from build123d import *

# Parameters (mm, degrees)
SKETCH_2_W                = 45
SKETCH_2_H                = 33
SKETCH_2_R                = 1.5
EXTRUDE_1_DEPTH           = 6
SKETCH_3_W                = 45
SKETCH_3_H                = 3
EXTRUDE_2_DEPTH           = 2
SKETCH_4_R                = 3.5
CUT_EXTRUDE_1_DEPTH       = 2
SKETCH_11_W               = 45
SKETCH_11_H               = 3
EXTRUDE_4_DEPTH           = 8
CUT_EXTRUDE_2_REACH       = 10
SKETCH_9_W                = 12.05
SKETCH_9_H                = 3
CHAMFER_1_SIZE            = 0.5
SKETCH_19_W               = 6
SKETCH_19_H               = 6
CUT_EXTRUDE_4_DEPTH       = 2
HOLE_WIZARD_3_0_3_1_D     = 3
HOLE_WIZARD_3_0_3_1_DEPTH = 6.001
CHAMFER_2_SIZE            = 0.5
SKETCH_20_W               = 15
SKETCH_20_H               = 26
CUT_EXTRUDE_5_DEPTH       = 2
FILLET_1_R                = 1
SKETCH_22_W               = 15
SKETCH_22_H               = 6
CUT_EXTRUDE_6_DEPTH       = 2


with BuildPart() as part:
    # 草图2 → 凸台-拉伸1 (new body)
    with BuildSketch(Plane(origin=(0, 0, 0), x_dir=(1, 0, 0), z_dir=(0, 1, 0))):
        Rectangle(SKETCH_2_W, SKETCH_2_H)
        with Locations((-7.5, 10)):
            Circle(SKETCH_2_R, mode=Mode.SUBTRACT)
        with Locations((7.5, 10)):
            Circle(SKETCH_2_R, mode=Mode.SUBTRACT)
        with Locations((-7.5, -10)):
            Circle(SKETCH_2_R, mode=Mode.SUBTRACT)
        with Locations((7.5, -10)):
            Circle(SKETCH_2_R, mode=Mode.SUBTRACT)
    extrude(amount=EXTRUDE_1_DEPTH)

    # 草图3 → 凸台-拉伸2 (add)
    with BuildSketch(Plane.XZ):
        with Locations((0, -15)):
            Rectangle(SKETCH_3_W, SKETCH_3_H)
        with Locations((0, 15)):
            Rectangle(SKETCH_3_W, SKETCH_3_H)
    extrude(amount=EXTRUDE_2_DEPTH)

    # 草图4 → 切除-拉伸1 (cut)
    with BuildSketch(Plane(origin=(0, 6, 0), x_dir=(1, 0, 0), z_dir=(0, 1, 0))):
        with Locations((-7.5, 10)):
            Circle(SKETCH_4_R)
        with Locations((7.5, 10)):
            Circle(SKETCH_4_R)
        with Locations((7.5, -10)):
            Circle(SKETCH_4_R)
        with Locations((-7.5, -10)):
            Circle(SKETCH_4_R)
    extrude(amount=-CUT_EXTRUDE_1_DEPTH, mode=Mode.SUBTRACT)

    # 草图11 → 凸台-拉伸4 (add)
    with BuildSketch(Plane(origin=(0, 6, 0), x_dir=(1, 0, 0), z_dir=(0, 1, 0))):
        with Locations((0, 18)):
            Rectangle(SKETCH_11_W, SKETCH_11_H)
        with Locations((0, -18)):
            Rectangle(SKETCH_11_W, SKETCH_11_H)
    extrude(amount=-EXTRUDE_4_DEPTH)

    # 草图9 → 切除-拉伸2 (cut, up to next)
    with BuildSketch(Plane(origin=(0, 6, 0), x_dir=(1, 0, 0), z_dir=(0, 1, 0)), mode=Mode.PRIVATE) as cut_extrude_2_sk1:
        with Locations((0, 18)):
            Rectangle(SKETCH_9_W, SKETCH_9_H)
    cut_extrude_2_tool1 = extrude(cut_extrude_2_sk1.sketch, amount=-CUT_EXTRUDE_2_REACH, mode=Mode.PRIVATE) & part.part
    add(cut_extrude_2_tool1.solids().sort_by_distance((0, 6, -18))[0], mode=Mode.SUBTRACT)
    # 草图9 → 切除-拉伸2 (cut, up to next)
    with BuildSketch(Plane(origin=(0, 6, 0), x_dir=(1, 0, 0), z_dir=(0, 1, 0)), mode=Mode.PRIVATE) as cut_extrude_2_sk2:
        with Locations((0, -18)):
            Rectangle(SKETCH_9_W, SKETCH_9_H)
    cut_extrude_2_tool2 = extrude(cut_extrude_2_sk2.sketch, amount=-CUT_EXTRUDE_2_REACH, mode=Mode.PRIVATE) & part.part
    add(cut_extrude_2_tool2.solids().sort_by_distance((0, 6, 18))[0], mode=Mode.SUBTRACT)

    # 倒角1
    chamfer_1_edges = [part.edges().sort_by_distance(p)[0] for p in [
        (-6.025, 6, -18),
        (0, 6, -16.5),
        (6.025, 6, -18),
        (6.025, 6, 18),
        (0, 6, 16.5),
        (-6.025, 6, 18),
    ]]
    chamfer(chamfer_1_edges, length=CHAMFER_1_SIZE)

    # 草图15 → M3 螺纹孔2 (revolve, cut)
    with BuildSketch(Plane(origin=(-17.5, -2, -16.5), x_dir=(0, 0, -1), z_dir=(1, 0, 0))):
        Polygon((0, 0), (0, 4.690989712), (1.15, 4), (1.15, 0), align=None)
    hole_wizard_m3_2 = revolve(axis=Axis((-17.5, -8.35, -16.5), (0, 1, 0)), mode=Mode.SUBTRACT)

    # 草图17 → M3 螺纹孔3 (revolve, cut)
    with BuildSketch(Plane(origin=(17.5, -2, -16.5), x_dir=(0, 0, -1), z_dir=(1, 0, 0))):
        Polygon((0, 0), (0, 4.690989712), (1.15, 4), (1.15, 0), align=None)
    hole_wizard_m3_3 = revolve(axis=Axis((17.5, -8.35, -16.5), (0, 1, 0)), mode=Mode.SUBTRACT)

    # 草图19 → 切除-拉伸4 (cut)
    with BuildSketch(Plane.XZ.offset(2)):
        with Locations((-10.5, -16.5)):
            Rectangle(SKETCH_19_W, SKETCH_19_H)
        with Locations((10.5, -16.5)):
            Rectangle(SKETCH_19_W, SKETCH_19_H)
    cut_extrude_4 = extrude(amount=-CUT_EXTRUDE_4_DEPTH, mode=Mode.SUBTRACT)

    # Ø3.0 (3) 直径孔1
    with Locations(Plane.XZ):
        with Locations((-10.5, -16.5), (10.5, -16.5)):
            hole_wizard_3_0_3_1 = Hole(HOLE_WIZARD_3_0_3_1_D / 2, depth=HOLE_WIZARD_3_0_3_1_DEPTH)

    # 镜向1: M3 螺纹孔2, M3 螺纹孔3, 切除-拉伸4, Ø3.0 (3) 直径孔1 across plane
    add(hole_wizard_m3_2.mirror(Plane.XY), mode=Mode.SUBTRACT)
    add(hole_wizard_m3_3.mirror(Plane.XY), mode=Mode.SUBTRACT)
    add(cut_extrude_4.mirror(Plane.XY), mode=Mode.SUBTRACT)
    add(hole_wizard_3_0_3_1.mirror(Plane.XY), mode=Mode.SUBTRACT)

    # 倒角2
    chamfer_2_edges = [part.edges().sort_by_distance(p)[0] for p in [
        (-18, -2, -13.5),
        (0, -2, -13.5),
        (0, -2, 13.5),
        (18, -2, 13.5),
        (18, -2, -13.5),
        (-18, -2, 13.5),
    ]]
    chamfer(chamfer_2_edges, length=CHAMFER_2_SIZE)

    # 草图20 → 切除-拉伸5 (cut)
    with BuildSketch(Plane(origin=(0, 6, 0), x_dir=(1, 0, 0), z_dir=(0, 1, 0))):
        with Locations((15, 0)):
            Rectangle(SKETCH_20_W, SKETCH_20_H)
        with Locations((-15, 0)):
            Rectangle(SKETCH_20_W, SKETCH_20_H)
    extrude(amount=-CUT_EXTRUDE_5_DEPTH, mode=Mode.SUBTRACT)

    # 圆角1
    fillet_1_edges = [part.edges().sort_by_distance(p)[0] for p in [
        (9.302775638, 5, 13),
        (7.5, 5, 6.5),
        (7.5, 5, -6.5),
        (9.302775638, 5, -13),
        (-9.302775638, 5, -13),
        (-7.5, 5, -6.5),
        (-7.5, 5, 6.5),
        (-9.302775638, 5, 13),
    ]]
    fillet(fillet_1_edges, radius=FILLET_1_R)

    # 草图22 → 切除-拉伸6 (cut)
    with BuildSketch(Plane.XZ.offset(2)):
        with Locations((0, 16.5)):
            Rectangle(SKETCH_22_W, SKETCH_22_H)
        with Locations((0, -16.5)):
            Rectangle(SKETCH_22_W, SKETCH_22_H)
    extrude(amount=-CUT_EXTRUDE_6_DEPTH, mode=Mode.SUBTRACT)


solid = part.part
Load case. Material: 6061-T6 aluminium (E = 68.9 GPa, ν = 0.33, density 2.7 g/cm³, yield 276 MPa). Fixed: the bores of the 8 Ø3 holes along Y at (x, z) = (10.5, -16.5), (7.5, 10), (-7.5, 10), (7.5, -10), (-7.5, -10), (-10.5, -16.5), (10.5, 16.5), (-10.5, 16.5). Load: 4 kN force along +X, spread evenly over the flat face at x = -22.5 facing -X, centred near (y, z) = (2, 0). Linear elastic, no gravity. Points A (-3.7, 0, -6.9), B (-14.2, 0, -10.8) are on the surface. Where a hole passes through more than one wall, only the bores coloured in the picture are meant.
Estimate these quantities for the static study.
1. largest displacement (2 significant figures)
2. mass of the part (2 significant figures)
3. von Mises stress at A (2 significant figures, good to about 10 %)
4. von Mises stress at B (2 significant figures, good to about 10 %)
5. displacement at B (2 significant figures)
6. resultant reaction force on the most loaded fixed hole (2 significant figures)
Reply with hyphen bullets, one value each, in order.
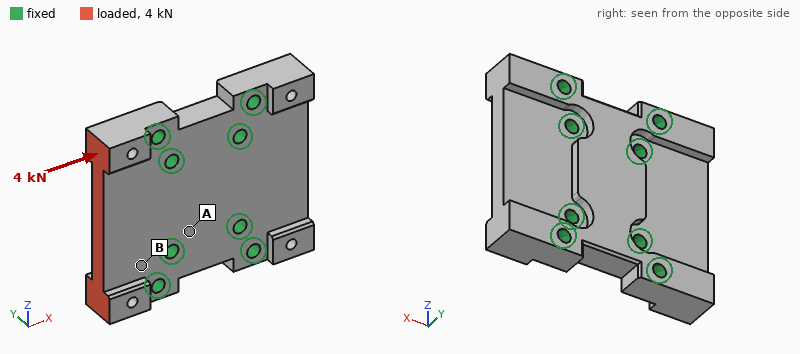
- 8.0 µm
- 23 g
- 9.8 MPa
- 24 MPa
- 2.6 µm
- 1.1 kN
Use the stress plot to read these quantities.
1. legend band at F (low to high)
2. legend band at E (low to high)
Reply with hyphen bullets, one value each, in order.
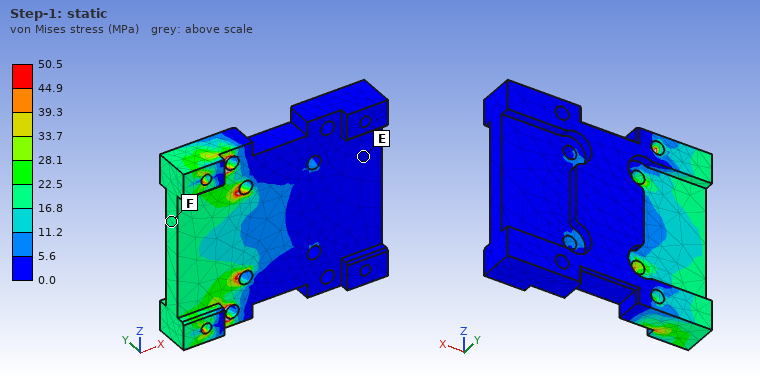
- 16.8 to 22.5 MPa
- 0.0 to 5.6 MPa
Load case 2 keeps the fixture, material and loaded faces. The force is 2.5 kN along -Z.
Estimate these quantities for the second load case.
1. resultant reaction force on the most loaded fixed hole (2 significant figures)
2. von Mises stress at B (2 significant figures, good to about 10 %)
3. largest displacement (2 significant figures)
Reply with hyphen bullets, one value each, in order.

- 1.1 kN
- 30 MPa
- 15 µm
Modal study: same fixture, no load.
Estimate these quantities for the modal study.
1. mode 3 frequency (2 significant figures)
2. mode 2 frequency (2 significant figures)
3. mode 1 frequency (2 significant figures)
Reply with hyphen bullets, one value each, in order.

- 28 kHz
- 20 kHz
- 20 kHz
